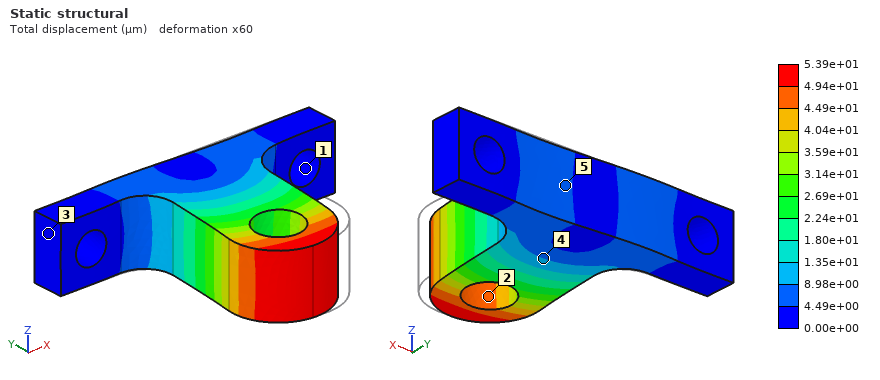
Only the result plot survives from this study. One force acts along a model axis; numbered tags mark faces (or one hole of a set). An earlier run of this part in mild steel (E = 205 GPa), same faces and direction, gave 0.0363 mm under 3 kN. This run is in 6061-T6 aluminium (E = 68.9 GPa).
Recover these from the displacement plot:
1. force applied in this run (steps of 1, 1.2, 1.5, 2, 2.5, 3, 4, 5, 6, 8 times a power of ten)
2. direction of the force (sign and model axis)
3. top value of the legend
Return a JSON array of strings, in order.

["1.5 kN", "-X", "5.39e+01 µm"]
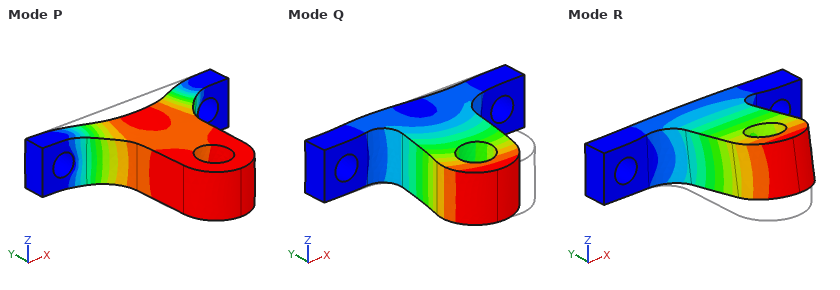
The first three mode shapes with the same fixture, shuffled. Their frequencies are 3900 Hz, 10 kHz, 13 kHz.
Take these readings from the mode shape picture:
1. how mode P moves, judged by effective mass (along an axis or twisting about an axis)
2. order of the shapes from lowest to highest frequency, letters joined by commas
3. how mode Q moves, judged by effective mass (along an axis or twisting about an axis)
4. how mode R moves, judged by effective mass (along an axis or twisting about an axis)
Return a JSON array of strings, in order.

["along Y", "R, Q, P", "along X", "along Z"]
